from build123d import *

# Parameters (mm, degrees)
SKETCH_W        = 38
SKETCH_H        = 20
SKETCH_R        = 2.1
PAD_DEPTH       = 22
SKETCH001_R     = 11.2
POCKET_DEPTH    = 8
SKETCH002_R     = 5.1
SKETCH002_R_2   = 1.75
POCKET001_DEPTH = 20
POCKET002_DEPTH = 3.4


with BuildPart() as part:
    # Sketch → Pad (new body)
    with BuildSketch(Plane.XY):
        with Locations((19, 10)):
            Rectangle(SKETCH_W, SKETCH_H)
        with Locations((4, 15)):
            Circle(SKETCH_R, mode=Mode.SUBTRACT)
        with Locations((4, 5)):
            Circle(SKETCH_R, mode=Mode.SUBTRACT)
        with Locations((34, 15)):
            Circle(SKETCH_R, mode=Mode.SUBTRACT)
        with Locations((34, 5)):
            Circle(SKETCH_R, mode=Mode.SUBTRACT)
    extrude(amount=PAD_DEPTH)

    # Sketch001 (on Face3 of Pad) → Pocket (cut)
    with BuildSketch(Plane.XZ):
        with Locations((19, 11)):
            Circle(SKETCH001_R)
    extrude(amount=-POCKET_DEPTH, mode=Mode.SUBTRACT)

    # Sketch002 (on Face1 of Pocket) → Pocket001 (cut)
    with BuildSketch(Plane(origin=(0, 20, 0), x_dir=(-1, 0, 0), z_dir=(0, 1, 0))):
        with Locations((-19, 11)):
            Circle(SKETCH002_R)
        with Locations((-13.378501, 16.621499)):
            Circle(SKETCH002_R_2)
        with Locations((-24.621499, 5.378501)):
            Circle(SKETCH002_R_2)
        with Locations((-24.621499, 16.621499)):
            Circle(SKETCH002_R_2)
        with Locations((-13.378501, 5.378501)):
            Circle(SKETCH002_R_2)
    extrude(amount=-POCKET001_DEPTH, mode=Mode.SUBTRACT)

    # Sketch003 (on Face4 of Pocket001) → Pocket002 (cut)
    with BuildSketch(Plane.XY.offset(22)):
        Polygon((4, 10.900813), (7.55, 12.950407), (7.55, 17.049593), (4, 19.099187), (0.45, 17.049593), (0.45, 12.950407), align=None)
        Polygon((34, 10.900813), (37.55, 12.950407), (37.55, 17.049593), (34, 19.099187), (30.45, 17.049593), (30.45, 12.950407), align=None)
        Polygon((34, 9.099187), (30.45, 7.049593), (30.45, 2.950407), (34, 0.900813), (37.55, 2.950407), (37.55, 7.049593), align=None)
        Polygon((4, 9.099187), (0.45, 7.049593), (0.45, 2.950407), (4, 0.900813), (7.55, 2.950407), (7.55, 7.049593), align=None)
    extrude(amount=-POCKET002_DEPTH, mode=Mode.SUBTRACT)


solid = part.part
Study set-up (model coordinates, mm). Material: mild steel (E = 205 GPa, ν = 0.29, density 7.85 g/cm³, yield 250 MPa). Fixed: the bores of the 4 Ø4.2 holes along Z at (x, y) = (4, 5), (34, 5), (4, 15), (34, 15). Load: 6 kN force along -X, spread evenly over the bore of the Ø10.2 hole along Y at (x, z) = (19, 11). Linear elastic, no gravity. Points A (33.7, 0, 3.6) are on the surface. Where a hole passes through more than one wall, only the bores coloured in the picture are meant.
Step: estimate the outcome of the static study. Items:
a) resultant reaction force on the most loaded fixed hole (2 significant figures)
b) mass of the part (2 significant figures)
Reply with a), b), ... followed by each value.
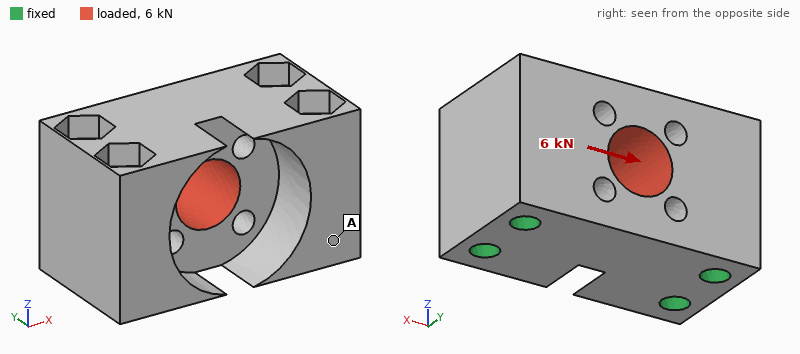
a) 2.4 kN
b) 82 g
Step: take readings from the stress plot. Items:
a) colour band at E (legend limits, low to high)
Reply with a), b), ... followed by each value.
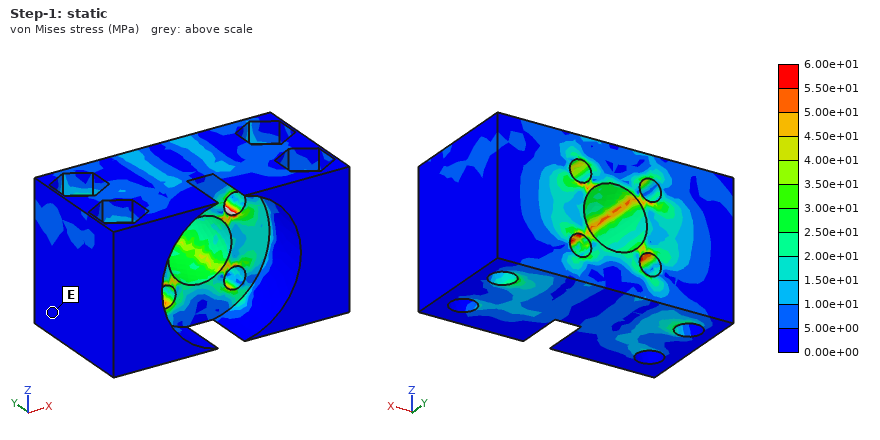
a) 0.00e+00 to 5.00e+00 MPa
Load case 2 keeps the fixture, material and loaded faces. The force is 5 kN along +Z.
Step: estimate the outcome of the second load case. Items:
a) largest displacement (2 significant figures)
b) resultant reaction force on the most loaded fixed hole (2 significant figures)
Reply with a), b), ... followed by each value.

a) 2.8 µm
b) 1.9 kN
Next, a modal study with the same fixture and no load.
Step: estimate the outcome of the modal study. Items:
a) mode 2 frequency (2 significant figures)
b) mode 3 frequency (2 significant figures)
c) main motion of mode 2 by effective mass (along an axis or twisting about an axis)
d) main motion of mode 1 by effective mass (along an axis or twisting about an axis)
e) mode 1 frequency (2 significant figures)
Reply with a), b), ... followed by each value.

a) 52 kHz
b) 56 kHz
c) along Z
d) along Y
e) 48 kHz
